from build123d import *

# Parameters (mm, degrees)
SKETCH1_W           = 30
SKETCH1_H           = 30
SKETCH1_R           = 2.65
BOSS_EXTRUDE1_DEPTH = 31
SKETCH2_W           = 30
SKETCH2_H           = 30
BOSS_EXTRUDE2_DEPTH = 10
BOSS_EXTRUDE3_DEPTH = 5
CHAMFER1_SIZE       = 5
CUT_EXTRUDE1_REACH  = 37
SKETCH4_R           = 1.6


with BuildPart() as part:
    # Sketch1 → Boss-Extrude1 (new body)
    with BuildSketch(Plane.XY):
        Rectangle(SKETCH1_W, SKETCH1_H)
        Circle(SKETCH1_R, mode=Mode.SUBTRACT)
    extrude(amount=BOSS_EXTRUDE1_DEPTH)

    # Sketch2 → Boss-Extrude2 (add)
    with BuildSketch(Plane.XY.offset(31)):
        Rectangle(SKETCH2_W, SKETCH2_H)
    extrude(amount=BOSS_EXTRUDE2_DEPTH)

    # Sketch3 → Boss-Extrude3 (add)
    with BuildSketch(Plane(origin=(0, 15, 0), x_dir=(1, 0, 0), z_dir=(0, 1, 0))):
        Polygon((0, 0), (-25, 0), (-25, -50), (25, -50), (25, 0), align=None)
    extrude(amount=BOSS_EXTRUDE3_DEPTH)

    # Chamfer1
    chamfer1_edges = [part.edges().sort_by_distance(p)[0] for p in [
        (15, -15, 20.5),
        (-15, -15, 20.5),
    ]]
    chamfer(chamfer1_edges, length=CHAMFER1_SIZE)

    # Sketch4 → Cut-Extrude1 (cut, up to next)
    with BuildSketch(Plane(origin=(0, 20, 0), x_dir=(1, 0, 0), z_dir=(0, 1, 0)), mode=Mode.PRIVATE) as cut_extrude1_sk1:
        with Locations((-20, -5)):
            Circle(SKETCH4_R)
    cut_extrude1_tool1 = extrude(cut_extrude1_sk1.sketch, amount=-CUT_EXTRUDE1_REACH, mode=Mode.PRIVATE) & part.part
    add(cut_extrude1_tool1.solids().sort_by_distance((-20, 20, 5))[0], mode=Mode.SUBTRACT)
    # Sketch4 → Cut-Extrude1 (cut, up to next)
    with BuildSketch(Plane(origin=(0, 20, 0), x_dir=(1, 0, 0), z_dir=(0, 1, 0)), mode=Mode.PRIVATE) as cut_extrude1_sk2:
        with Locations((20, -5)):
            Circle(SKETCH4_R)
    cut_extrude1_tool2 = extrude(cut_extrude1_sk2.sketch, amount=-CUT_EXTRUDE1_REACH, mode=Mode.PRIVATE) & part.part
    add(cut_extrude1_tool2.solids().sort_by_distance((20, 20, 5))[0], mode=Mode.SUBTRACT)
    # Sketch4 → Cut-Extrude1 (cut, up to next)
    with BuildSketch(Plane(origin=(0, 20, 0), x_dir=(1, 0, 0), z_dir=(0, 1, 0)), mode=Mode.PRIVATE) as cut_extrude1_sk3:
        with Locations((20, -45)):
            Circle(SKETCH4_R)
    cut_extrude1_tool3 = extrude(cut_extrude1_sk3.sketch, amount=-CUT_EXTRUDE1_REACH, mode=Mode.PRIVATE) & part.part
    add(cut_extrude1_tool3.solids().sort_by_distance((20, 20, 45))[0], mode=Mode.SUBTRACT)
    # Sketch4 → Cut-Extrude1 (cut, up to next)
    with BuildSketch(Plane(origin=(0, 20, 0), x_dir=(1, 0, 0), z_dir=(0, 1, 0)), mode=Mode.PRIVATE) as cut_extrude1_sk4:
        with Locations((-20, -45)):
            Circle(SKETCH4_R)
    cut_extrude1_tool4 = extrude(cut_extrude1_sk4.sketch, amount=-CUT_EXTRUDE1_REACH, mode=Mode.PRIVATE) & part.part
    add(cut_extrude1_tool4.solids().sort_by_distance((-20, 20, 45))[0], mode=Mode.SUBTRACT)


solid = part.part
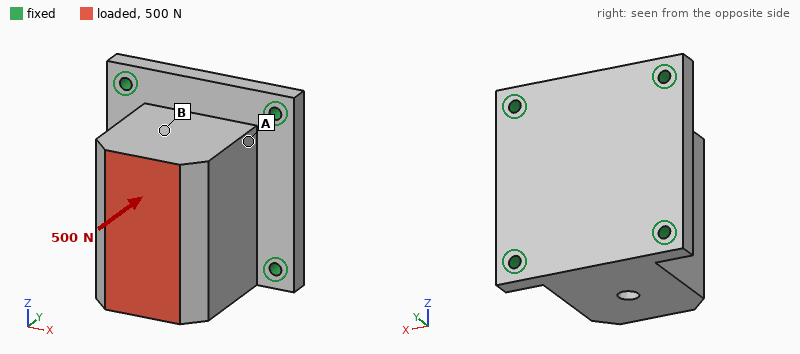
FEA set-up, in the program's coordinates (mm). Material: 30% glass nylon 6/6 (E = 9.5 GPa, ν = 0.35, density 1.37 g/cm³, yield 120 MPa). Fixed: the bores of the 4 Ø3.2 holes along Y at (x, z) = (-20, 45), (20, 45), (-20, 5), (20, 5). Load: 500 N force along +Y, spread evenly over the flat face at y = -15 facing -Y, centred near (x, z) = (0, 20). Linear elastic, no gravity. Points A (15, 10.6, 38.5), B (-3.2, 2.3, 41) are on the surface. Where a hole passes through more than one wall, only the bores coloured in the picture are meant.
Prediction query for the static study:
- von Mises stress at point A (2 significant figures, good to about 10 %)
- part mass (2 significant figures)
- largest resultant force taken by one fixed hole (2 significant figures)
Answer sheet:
2.5 MPa
65 g
160 N
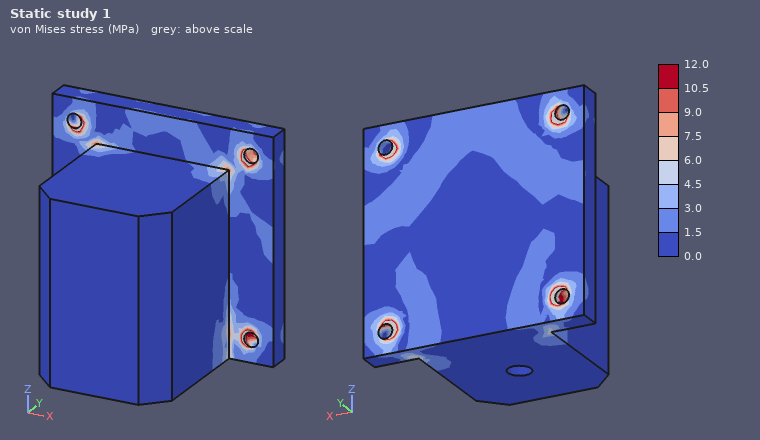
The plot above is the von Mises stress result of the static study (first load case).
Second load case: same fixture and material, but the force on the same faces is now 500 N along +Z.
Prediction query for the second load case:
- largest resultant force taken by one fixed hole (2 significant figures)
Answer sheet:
270 N
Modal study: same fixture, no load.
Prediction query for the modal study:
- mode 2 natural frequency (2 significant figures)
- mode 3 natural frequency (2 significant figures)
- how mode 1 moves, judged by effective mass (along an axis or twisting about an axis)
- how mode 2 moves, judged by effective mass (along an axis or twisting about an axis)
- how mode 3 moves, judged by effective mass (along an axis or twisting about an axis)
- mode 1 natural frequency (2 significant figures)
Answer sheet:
3700 Hz
4400 Hz
along Z
along X
along Y
3400 Hz
